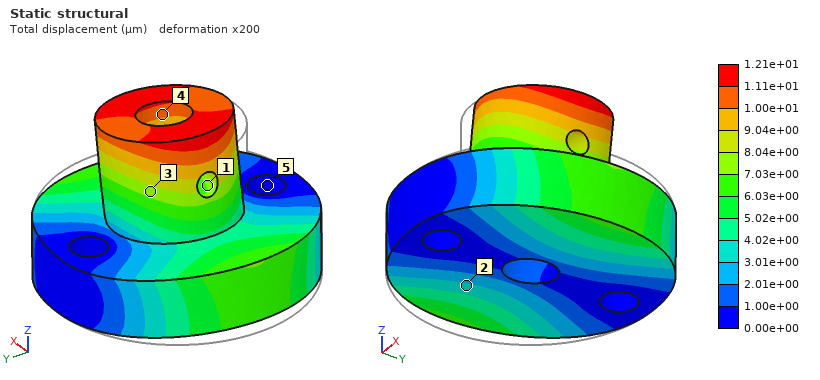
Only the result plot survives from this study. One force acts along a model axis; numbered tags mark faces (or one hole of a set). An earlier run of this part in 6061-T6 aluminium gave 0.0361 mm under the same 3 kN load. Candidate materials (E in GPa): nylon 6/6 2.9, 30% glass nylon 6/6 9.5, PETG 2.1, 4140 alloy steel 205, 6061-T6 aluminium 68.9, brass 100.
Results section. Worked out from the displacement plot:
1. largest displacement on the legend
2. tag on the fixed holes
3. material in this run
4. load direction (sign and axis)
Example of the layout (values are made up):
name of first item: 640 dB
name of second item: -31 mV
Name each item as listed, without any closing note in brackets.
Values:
largest displacement on the legend: 1.21e+01 µm
tag on the fixed holes: 5
material in this run: 4140 alloy steel
load direction: +X
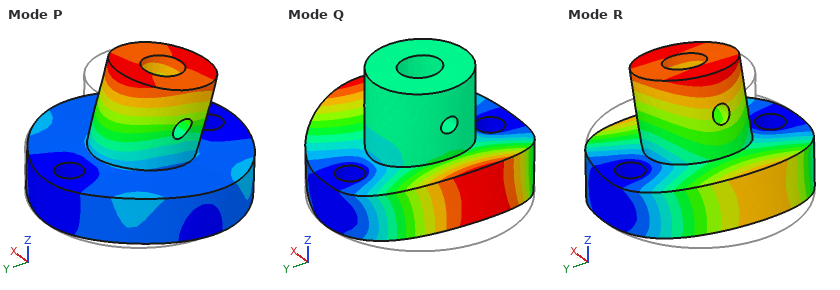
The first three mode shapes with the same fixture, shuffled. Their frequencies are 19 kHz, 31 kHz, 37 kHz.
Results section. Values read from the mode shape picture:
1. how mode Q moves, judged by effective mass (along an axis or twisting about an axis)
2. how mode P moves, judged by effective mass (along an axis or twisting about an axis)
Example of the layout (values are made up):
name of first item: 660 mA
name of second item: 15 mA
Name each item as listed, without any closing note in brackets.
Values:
how mode Q moves, judged by effective mass: along Z
how mode P moves, judged by effective mass: along Y
